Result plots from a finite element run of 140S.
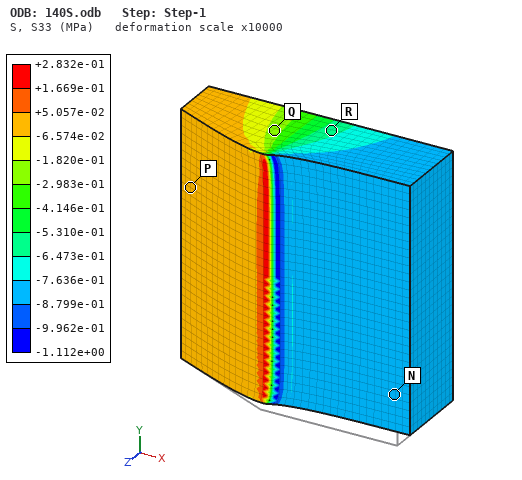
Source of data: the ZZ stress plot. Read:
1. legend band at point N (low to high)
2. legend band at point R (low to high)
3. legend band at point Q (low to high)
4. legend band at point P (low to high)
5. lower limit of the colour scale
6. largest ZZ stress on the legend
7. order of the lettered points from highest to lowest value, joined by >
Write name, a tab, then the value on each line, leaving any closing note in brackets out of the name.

legend band at point N	-8.799e-01 to -7.636e-01 MPa
legend band at point R	-6.473e-01 to -5.310e-01 MPa
legend band at point Q	-2.983e-01 to -1.820e-01 MPa
legend band at point P	-6.574e-02 to +5.057e-02 MPa
lower limit of the colour scale	-1.112e+00 MPa
largest ZZ stress on the legend	+2.832e-01 MPa
order of the lettered points from highest to lowest value, joined by >	P > Q > R > N
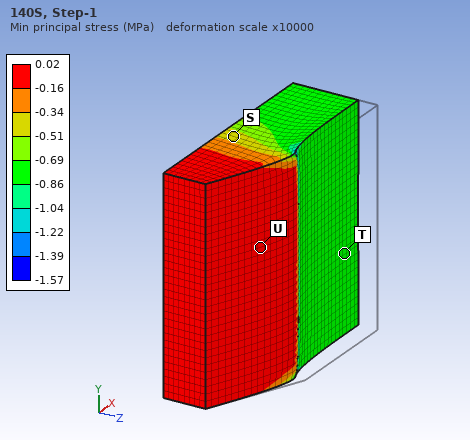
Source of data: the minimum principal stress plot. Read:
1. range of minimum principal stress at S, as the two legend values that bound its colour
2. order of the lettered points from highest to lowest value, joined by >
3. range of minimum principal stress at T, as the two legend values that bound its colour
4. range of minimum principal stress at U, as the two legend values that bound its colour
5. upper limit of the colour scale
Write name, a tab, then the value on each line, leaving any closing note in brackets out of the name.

range of minimum principal stress at S, as the two legend values that bound its colour	-0.51 to -0.34 MPa
order of the lettered points from highest to lowest value, joined by >	U > S > T
range of minimum principal stress at T, as the two legend values that bound its colour	-0.86 to -0.69 MPa
range of minimum principal stress at U, as the two legend values that bound its colour	-0.16 to 0.02 MPa
upper limit of the colour scale	0.02 MPa
